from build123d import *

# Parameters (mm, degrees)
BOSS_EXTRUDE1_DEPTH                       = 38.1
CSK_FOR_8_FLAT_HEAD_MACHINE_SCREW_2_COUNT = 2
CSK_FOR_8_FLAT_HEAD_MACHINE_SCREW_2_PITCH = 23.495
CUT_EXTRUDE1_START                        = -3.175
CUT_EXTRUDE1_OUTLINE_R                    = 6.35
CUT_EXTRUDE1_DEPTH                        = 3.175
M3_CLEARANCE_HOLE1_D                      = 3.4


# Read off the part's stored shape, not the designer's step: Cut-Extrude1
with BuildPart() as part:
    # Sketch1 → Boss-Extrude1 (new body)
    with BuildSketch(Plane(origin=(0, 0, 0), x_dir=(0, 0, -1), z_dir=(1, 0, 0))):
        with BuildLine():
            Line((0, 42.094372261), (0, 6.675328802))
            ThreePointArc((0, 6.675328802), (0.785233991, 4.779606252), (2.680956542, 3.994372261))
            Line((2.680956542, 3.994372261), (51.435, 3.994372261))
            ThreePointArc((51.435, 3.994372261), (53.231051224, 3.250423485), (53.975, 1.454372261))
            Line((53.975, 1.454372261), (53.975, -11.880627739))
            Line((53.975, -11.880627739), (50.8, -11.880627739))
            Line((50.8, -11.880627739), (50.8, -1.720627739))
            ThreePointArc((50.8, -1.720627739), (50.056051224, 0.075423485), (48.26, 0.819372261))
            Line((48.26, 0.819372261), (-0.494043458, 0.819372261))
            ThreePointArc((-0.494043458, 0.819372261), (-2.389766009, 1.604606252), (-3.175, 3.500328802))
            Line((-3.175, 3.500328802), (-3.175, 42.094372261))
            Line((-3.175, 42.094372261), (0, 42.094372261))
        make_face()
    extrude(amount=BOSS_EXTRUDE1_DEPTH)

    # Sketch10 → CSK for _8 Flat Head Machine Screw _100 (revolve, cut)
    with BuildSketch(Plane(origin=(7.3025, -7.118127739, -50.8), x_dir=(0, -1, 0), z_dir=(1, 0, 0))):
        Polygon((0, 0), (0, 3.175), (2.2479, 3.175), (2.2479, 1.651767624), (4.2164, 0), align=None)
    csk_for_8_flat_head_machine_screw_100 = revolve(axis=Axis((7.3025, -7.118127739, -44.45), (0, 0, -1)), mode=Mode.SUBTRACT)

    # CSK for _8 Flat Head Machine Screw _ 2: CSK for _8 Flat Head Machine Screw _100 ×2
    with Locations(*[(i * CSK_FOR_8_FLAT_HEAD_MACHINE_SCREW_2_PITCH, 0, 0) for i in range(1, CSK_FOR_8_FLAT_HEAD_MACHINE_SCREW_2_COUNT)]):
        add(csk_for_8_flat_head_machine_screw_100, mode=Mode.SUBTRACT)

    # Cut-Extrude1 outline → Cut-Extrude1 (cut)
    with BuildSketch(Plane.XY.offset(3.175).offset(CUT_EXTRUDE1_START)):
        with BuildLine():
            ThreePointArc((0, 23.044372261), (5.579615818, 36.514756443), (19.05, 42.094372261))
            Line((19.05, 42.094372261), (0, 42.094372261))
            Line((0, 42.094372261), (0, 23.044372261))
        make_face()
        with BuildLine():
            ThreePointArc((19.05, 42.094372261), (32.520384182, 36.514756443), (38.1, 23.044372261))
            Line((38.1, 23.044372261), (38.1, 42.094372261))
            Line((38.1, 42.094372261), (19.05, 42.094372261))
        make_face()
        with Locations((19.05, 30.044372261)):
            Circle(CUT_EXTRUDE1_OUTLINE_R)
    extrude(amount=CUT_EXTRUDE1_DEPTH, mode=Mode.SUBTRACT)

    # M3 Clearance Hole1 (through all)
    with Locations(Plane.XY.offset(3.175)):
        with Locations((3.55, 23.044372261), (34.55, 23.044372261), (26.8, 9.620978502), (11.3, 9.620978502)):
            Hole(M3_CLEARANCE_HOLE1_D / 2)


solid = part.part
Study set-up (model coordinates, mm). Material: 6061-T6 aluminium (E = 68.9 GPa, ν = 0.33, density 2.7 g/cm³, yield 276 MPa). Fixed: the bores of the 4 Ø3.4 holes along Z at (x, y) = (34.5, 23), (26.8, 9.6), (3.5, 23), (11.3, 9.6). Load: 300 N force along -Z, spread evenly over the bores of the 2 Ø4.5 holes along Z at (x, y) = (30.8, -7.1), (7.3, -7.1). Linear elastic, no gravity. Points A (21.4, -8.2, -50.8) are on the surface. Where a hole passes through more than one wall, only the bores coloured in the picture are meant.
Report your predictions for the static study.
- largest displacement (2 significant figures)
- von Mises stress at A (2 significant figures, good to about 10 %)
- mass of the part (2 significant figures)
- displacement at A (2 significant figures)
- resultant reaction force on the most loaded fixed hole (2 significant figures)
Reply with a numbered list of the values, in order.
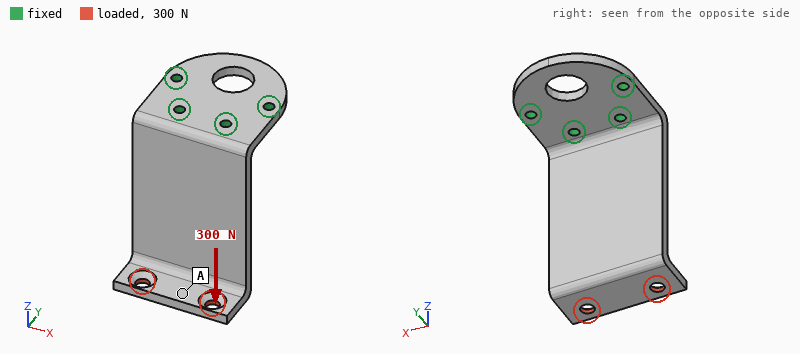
1. 0.82 mm
2. 10 MPa
3. 32 g
4. 0.72 mm
5. 200 N
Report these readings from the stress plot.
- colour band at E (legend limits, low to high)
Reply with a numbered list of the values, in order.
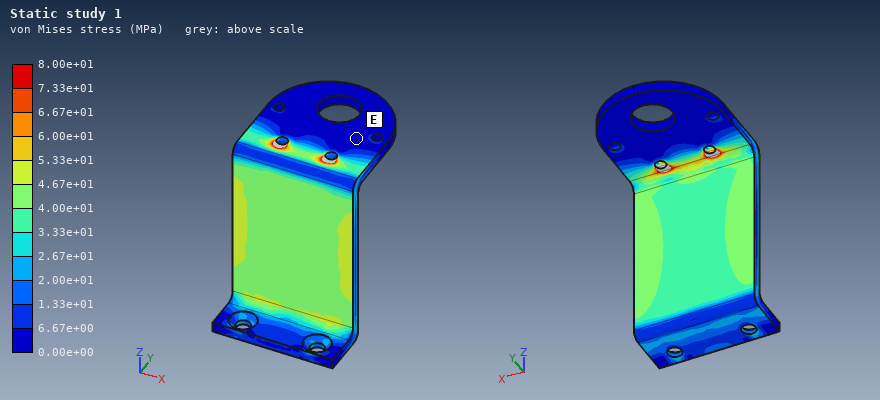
1. 0.00e+00 to 6.67e+00 MPa
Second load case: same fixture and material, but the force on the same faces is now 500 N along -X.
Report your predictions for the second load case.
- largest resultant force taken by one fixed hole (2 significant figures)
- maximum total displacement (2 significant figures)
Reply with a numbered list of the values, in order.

1. 1.5 kN
2. 0.51 mm
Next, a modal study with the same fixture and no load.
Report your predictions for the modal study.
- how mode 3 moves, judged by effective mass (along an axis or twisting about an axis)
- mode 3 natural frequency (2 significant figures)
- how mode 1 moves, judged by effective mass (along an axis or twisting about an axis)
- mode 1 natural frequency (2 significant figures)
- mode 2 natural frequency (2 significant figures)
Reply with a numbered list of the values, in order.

1. along X
2. 2200 Hz
3. along Y
4. 570 Hz
5. 2000 Hz
